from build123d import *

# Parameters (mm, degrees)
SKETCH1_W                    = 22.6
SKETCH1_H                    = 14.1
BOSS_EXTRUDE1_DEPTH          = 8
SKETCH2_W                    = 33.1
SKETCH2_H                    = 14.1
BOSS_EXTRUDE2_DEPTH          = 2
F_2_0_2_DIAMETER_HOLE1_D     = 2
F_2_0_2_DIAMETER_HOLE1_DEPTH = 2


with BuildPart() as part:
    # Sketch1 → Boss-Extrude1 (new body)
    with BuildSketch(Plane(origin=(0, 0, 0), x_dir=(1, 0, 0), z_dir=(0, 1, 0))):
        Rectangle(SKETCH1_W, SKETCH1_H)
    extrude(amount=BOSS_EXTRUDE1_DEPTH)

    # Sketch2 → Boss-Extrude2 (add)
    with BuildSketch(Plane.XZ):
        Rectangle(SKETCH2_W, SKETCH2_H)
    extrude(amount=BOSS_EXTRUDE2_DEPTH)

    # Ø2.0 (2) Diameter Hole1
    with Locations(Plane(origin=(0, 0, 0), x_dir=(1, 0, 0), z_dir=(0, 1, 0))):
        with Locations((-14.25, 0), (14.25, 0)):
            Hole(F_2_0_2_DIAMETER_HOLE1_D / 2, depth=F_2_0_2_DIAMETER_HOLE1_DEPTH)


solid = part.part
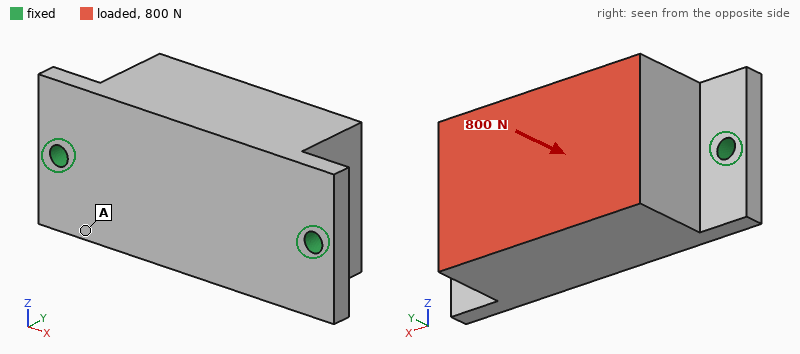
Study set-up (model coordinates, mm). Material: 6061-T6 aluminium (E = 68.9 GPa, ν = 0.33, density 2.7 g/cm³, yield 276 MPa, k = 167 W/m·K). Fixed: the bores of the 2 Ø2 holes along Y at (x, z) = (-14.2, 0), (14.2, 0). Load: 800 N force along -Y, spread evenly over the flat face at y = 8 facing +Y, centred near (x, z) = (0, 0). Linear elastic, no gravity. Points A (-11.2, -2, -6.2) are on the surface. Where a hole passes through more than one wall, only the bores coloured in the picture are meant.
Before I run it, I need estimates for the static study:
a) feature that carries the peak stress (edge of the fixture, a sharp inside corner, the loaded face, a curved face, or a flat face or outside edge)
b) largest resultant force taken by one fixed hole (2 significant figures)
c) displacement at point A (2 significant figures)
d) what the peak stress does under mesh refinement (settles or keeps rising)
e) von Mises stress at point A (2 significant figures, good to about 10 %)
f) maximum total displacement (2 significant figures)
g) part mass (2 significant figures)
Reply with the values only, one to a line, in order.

edge of the fixture
450 N
9.1 µm
keeps rising
23 MPa
11 µm
9.4 g
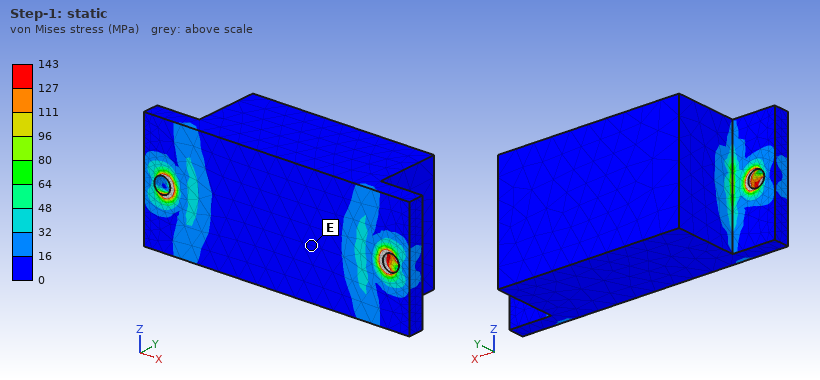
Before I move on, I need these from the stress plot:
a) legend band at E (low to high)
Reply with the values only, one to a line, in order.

0 to 16 MPa
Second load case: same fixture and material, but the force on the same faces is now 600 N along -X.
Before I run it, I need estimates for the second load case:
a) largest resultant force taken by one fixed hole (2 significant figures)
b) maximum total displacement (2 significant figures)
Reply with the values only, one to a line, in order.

370 N
6.8 µm
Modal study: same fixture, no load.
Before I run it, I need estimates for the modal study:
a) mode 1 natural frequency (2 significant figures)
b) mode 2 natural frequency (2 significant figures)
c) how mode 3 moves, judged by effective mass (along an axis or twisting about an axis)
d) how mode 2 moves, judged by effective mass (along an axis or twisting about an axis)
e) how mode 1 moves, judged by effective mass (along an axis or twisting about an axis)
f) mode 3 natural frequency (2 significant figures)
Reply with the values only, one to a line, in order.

5800 Hz
15 kHz
along X
along Y
along Z
23 kHz
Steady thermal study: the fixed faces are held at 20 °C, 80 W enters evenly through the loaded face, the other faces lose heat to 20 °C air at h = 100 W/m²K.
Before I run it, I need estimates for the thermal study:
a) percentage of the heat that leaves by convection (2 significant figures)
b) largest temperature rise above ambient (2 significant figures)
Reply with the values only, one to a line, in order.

8.1 %
67 K
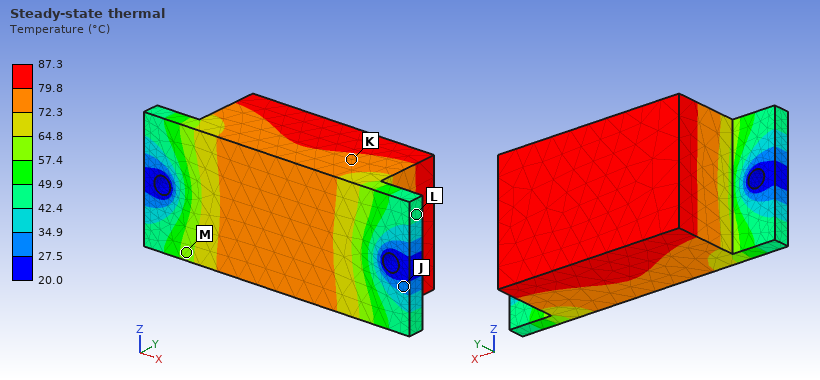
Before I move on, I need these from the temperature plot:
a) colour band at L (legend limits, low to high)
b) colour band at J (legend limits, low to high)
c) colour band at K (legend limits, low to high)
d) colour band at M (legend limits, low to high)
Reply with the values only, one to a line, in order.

42.4 to 49.9 °C
27.5 to 34.9 °C
72.3 to 79.8 °C
57.4 to 64.8 °C
